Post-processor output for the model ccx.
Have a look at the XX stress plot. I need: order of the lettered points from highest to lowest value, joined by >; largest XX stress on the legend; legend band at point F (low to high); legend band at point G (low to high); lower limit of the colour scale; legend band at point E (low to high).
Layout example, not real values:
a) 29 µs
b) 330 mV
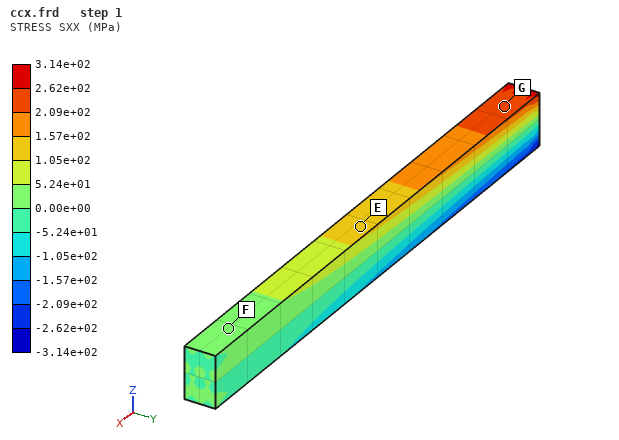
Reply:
a) G > E > F
b) 3.14e+02 MPa
c) 0.00e+00 to 5.24e+01 MPa
d) 2.09e+02 to 2.62e+02 MPa
e) -3.14e+02 MPa
f) 1.05e+02 to 1.57e+02 MPa
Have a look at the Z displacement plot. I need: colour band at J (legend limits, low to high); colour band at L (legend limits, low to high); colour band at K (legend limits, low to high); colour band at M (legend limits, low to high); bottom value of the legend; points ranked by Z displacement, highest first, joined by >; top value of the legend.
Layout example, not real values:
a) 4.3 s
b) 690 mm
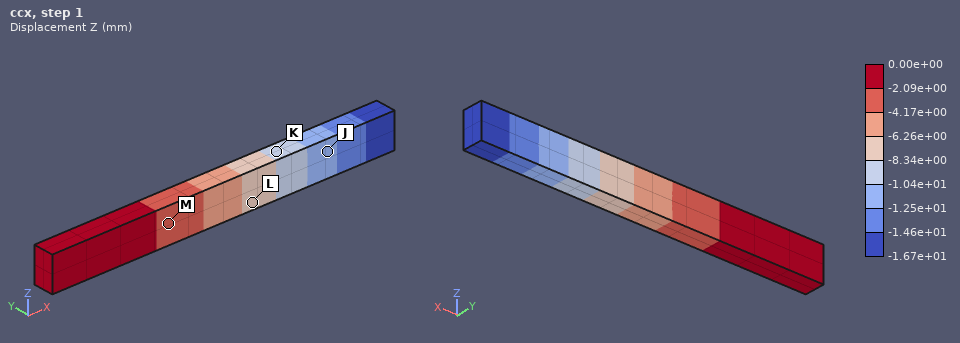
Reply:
a) -1.25e+01 to -1.04e+01 mm
b) -8.34e+00 to -6.26e+00 mm
c) -1.04e+01 to -8.34e+00 mm
d) -4.17e+00 to -2.09e+00 mm
e) -1.67e+01 mm
f) M > L > K > J
g) 0.00e+00 mm
